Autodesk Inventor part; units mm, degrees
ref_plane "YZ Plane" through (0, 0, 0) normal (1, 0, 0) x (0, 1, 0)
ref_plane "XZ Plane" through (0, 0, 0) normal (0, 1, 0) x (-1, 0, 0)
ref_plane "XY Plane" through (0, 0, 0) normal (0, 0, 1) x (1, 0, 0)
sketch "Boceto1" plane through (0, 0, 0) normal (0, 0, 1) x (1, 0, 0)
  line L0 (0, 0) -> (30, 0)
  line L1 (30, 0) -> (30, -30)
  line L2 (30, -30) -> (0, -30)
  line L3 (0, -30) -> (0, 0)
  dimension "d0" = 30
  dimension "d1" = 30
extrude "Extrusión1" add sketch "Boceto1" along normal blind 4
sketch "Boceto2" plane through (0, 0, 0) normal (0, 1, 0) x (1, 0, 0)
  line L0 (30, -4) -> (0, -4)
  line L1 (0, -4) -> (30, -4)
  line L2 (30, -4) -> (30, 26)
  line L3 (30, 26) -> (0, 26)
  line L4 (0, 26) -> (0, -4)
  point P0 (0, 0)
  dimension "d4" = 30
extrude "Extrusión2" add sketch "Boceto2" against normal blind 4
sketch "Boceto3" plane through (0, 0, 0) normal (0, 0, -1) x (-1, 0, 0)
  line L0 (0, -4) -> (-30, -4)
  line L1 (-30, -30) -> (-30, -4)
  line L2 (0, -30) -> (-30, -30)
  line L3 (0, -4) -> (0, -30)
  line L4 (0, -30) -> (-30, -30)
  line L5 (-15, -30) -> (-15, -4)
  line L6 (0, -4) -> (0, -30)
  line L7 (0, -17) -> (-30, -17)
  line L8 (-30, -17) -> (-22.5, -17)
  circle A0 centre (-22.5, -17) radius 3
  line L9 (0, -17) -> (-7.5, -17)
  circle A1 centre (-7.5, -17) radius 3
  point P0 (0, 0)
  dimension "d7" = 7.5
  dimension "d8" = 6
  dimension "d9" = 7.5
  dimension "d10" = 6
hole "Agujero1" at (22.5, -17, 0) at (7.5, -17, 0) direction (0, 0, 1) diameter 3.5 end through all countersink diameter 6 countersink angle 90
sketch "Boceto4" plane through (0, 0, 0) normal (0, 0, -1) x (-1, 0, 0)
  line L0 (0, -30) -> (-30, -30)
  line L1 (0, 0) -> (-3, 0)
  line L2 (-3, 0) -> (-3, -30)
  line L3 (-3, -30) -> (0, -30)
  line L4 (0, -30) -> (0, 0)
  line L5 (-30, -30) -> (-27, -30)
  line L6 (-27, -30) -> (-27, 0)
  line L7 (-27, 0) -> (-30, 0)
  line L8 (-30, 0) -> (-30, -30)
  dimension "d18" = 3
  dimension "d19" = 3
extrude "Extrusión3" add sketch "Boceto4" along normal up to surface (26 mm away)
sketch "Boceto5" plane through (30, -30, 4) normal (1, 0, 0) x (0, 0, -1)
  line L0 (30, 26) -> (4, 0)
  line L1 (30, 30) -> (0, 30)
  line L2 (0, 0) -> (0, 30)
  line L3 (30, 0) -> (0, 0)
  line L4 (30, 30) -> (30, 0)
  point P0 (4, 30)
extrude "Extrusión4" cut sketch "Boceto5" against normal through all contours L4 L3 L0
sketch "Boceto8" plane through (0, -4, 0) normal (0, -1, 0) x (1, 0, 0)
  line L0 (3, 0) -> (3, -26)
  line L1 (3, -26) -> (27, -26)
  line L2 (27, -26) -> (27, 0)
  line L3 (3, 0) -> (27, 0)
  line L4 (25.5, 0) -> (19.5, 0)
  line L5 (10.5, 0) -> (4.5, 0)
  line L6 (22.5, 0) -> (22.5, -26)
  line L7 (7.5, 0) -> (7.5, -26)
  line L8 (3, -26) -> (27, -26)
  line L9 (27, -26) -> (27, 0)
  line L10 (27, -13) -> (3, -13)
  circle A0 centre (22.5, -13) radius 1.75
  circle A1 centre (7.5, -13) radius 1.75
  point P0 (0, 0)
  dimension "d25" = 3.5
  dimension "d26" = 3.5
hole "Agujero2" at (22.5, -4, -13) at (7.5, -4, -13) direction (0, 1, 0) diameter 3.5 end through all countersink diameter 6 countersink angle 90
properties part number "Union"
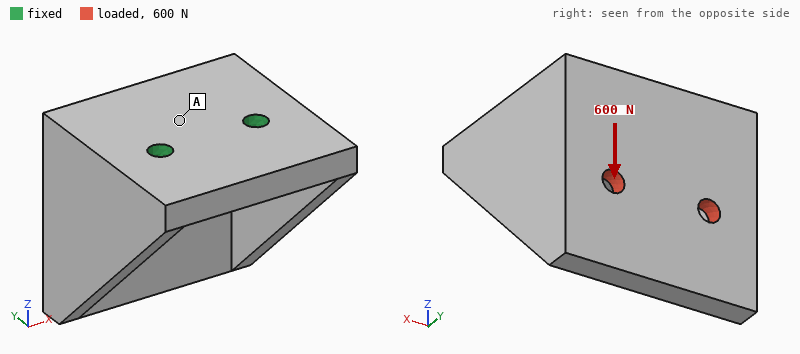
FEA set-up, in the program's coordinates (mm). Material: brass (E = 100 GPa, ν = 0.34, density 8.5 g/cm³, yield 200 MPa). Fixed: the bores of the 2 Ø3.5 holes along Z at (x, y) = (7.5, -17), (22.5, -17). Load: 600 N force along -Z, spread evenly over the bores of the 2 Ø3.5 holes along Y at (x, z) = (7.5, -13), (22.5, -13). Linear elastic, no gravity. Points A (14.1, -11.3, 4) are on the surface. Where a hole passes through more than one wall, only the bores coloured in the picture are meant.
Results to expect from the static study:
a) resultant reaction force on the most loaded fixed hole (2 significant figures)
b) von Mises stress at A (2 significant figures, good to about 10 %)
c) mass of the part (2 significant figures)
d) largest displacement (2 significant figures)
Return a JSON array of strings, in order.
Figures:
["300 N", "27 MPa", "73 g", "73 µm"]
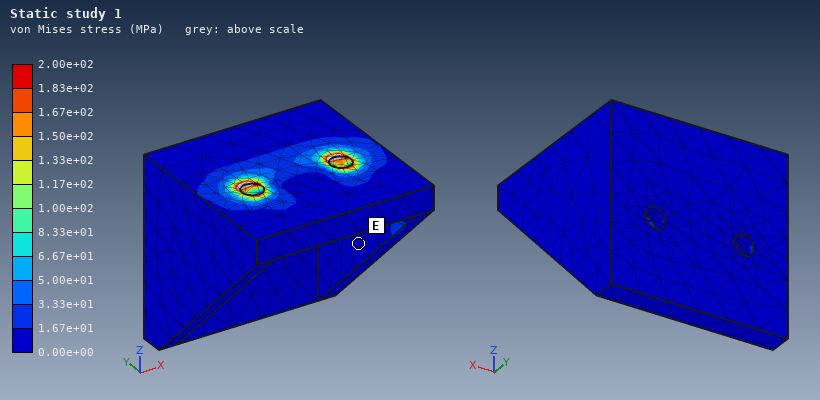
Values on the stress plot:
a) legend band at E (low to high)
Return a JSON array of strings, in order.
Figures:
["0.00e+00 to 1.67e+01 MPa"]
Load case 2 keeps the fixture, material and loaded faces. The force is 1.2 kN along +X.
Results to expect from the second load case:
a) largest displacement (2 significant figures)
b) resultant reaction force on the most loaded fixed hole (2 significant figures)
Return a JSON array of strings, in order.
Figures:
["0.10 mm", "1.5 kN"]
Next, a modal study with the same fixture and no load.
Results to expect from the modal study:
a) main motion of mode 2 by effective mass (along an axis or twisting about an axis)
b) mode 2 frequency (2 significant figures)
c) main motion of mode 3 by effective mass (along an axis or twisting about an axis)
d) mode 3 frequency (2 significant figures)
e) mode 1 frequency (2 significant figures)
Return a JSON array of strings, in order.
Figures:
["along X", "3100 Hz", "along X", "8100 Hz", "2300 Hz"]
